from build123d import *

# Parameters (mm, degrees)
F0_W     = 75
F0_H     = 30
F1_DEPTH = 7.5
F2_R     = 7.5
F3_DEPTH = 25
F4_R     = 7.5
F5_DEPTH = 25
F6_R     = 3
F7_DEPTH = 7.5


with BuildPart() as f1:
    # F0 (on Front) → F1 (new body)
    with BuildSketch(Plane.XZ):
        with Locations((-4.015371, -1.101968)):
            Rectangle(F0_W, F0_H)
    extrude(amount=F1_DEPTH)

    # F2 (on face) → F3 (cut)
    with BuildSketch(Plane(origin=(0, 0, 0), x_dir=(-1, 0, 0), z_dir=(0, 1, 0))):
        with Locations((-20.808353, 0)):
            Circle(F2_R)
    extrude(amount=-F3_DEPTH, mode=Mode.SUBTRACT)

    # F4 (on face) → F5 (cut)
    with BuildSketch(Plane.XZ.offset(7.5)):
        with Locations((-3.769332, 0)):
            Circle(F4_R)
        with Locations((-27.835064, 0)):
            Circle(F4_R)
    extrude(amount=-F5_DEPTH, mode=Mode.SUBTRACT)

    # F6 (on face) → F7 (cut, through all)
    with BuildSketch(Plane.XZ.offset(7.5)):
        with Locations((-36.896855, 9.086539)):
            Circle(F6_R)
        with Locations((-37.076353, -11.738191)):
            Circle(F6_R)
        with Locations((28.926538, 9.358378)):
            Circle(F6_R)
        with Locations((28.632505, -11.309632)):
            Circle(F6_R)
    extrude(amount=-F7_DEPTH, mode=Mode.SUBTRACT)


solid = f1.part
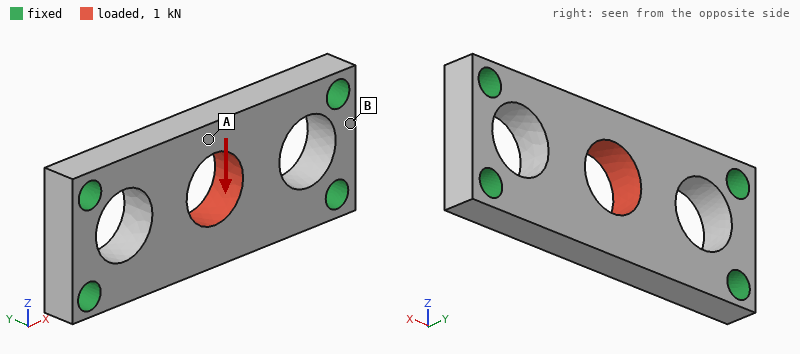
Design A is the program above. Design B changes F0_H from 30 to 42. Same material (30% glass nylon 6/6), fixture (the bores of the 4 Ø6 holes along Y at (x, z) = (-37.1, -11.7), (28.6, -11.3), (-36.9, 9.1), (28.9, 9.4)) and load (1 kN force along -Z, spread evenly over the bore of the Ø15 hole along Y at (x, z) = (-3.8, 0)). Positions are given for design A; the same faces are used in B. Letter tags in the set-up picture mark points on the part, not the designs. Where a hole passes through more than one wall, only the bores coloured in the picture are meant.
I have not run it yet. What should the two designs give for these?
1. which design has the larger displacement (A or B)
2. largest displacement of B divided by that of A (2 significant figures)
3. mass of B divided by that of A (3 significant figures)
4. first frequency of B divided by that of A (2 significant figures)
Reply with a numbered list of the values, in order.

1. A
2. 0.61
3. 1.56
4. 0.99
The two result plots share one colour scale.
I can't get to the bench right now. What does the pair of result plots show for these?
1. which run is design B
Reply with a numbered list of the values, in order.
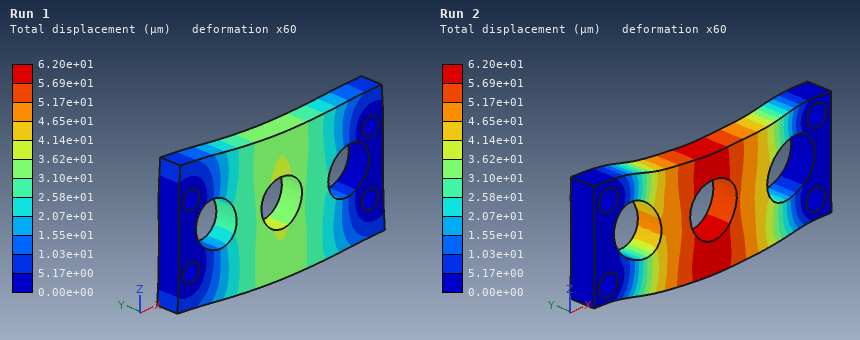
1. Run 1
